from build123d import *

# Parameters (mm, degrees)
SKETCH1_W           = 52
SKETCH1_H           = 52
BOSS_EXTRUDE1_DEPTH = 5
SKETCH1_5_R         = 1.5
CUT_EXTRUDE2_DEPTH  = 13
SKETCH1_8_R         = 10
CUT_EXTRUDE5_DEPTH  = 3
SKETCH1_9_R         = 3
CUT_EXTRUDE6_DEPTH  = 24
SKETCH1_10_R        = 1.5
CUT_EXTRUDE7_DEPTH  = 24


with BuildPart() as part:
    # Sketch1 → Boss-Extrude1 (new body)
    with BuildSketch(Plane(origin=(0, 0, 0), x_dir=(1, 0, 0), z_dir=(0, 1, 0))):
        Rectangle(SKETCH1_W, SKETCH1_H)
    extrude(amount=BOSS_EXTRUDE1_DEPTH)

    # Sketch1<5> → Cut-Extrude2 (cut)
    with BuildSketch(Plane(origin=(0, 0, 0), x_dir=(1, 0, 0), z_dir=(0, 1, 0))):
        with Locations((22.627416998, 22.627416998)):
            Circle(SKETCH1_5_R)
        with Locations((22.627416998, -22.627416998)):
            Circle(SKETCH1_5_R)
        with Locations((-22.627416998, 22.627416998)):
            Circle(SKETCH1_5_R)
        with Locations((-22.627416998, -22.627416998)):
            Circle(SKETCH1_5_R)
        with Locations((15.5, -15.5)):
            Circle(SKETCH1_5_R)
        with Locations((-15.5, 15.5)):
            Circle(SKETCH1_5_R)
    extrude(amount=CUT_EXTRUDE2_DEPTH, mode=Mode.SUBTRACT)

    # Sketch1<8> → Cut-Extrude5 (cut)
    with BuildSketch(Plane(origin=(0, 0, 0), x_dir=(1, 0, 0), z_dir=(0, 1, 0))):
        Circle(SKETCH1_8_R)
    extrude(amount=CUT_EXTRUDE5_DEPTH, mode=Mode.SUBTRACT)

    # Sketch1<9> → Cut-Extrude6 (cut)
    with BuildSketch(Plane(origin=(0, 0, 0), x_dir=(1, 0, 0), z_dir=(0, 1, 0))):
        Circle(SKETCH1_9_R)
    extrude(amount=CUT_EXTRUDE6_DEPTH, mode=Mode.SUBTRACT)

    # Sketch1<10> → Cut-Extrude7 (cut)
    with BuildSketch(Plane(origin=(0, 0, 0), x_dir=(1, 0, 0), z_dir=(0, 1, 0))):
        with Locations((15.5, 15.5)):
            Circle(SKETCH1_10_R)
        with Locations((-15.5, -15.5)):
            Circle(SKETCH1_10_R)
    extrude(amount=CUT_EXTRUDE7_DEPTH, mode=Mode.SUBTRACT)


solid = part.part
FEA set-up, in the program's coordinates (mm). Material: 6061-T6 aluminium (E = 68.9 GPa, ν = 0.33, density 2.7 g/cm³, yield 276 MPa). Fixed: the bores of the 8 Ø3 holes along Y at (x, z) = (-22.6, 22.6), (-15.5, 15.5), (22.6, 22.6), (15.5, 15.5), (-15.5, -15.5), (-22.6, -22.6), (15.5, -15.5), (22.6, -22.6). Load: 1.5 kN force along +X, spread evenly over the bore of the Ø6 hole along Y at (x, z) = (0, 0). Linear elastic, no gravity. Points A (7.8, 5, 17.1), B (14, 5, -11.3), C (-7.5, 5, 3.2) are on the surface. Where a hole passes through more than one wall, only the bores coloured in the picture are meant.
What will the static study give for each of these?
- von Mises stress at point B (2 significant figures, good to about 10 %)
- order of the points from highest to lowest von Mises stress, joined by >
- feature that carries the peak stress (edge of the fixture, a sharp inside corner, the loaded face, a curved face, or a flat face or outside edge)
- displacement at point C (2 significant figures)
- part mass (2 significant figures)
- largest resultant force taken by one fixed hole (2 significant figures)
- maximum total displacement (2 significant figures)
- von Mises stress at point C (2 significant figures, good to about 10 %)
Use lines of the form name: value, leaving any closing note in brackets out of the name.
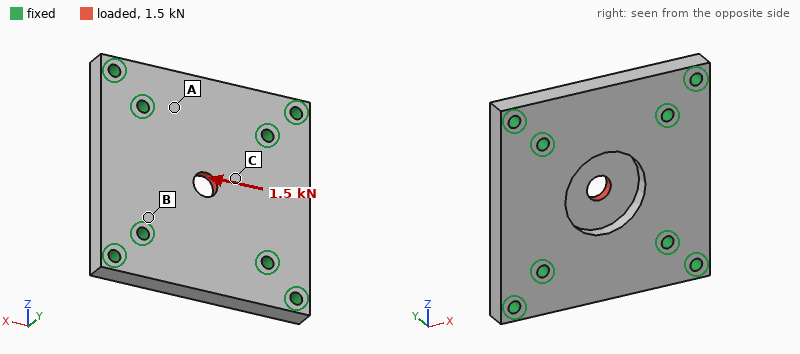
von Mises stress at point B: 10 MPa
order of the points from highest to lowest von Mises stress, joined by >: C > B > A
feature that carries the peak stress: the loaded face
displacement at point C: 3.6 µm
part mass: 33 g
largest resultant force taken by one fixed hole: 350 N
maximum total displacement: 5.8 µm
von Mises stress at point C: 18 MPa
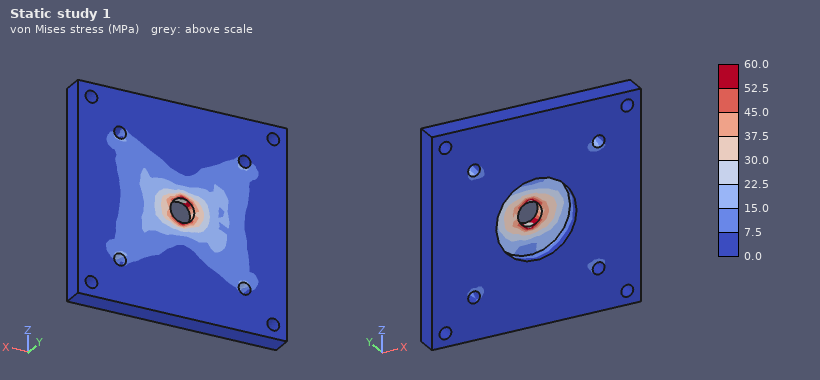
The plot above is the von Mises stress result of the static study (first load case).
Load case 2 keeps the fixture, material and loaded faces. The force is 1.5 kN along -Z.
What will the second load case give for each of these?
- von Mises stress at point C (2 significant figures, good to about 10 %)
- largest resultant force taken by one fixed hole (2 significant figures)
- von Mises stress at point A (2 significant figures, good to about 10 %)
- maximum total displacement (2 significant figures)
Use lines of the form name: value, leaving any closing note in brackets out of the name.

von Mises stress at point C: 12 MPa
largest resultant force taken by one fixed hole: 350 N
von Mises stress at point A: 7.1 MPa
maximum total displacement: 5.8 µm
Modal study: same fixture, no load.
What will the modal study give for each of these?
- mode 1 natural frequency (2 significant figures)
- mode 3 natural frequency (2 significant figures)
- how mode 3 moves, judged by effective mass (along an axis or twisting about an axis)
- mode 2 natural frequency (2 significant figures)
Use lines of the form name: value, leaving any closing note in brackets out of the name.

mode 1 natural frequency: 19 kHz
mode 3 natural frequency: 21 kHz
how mode 3 moves, judged by effective mass: twisting about X
mode 2 natural frequency: 19 kHz
